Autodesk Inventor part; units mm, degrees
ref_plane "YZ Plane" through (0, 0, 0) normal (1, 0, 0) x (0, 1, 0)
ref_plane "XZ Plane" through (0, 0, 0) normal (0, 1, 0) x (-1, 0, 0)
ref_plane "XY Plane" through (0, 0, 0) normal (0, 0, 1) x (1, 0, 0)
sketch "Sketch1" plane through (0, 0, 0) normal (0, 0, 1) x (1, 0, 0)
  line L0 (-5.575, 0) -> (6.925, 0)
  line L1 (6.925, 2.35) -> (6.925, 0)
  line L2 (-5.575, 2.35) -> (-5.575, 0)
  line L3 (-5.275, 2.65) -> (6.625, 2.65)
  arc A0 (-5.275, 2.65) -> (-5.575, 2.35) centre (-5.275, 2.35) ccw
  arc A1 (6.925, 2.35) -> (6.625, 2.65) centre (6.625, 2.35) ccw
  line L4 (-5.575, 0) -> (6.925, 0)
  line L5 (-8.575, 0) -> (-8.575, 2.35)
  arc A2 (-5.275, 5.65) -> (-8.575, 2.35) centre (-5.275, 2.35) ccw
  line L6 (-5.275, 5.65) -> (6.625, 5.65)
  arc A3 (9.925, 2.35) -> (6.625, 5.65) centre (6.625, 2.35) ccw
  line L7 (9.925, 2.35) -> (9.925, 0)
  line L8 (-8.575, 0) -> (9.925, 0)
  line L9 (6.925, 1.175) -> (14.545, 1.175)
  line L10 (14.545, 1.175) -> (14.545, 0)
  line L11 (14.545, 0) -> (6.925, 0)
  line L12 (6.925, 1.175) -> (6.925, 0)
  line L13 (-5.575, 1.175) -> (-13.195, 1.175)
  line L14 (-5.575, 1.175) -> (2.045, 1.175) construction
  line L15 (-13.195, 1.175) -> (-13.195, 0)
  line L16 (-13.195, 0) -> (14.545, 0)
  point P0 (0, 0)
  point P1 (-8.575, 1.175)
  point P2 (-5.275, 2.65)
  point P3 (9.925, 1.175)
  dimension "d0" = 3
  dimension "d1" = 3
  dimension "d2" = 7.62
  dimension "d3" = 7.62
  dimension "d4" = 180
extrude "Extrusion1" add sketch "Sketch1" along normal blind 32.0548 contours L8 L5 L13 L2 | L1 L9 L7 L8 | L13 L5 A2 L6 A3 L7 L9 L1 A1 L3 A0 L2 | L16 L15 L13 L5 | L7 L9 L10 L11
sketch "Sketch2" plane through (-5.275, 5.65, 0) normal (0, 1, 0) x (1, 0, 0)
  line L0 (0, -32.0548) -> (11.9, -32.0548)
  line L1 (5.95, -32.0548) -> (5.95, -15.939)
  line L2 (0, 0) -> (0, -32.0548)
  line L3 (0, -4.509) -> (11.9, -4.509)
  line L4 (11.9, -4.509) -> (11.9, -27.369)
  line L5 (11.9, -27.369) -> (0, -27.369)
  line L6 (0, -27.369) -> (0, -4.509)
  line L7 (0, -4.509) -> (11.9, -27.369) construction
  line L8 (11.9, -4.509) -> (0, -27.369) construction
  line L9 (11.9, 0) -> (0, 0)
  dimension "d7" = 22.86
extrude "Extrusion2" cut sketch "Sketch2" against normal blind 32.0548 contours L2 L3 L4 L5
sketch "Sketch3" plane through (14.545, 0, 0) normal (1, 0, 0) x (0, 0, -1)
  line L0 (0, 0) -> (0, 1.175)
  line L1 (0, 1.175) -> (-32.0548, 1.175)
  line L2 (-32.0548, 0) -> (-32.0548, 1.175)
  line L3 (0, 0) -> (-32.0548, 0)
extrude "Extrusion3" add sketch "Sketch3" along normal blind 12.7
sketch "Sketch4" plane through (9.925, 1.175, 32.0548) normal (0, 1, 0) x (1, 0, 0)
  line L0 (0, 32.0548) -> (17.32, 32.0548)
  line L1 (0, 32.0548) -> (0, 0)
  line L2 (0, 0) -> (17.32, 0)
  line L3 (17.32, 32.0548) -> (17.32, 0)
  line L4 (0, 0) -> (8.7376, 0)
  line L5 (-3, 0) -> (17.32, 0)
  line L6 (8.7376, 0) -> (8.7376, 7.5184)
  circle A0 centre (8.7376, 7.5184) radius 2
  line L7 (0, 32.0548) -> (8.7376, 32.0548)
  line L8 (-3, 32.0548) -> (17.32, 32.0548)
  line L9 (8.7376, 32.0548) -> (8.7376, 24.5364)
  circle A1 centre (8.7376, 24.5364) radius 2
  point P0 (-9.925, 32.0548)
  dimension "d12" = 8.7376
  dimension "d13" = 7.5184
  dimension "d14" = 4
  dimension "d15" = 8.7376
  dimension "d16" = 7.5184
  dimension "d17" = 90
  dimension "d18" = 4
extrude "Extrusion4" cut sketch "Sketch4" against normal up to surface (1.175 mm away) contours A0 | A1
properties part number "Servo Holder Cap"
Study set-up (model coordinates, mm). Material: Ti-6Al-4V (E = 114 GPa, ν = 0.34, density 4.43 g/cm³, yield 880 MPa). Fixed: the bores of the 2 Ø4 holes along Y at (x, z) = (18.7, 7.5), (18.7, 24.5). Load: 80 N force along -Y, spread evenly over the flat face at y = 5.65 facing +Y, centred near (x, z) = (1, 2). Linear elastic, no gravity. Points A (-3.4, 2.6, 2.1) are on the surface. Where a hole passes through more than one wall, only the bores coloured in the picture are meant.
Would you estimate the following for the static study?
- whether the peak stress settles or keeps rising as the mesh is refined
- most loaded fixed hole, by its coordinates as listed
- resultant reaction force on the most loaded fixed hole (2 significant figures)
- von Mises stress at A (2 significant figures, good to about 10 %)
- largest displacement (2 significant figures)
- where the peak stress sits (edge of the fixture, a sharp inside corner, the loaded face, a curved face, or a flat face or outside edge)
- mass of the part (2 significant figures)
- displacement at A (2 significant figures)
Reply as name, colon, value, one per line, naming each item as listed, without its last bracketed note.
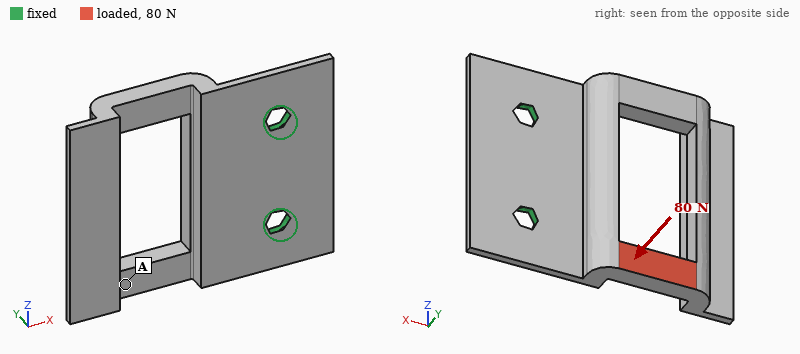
whether the peak stress settles or keeps rising as the mesh is refined: keeps rising
most loaded fixed hole, by its coordinates as listed: (18.7, 7.5)
resultant reaction force on the most loaded fixed hole: 93 N
von Mises stress at A: 26 MPa
largest displacement: 0.54 mm
where the peak stress sits: edge of the fixture
mass of the part: 9.4 g
displacement at A: 0.35 mm
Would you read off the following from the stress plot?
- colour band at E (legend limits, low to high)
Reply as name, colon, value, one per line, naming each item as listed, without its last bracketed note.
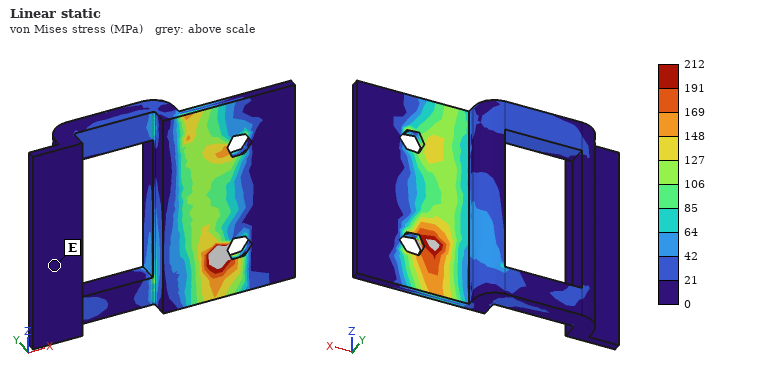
colour band at E: 0 to 21 MPa
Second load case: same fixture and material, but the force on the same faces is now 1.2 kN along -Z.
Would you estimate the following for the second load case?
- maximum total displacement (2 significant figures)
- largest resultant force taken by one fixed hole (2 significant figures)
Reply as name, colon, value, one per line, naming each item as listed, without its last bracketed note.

maximum total displacement: 0.24 mm
largest resultant force taken by one fixed hole: 1.3 kN
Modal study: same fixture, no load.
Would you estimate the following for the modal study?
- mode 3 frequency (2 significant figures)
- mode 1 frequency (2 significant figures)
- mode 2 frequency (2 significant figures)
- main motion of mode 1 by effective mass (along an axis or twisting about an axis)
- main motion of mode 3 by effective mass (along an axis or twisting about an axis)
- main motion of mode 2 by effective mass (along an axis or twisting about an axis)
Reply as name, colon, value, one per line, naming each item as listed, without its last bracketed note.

mode 3 frequency: 5700 Hz
mode 1 frequency: 920 Hz
mode 2 frequency: 3100 Hz
main motion of mode 1 by effective mass: along Y
main motion of mode 3 by effective mass: along Z
main motion of mode 2 by effective mass: twisting about X
